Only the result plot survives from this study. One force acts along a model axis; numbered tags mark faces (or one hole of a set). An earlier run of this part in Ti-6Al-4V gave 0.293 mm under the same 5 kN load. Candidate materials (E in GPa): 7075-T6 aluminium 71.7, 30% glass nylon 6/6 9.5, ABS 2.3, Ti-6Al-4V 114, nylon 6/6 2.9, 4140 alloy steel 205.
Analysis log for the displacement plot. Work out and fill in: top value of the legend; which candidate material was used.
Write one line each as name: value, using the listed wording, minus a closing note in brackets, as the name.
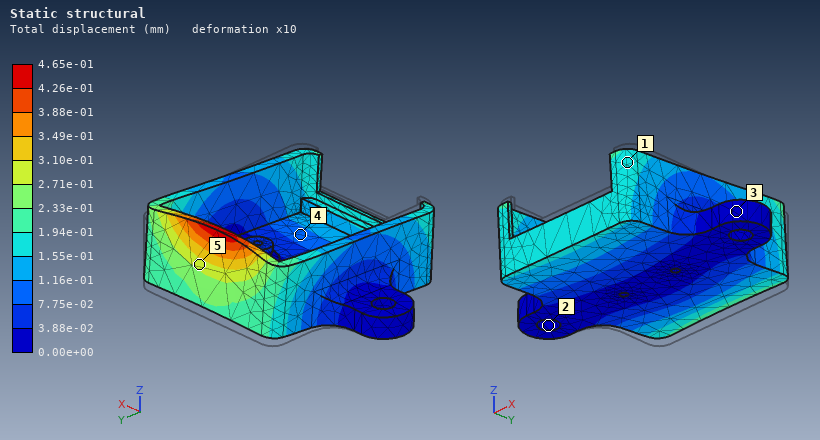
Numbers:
top value of the legend: 4.65e-01 mm
which candidate material was used: 7075-T6 aluminium
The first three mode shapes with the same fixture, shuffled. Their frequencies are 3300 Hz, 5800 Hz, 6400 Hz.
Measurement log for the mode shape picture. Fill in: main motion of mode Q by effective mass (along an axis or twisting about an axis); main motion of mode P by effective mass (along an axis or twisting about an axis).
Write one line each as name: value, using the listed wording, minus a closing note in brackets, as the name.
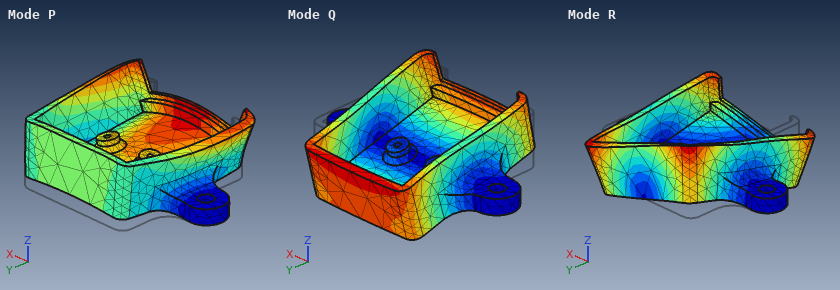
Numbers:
main motion of mode Q by effective mass: twisting about X
main motion of mode P by effective mass: along Z
